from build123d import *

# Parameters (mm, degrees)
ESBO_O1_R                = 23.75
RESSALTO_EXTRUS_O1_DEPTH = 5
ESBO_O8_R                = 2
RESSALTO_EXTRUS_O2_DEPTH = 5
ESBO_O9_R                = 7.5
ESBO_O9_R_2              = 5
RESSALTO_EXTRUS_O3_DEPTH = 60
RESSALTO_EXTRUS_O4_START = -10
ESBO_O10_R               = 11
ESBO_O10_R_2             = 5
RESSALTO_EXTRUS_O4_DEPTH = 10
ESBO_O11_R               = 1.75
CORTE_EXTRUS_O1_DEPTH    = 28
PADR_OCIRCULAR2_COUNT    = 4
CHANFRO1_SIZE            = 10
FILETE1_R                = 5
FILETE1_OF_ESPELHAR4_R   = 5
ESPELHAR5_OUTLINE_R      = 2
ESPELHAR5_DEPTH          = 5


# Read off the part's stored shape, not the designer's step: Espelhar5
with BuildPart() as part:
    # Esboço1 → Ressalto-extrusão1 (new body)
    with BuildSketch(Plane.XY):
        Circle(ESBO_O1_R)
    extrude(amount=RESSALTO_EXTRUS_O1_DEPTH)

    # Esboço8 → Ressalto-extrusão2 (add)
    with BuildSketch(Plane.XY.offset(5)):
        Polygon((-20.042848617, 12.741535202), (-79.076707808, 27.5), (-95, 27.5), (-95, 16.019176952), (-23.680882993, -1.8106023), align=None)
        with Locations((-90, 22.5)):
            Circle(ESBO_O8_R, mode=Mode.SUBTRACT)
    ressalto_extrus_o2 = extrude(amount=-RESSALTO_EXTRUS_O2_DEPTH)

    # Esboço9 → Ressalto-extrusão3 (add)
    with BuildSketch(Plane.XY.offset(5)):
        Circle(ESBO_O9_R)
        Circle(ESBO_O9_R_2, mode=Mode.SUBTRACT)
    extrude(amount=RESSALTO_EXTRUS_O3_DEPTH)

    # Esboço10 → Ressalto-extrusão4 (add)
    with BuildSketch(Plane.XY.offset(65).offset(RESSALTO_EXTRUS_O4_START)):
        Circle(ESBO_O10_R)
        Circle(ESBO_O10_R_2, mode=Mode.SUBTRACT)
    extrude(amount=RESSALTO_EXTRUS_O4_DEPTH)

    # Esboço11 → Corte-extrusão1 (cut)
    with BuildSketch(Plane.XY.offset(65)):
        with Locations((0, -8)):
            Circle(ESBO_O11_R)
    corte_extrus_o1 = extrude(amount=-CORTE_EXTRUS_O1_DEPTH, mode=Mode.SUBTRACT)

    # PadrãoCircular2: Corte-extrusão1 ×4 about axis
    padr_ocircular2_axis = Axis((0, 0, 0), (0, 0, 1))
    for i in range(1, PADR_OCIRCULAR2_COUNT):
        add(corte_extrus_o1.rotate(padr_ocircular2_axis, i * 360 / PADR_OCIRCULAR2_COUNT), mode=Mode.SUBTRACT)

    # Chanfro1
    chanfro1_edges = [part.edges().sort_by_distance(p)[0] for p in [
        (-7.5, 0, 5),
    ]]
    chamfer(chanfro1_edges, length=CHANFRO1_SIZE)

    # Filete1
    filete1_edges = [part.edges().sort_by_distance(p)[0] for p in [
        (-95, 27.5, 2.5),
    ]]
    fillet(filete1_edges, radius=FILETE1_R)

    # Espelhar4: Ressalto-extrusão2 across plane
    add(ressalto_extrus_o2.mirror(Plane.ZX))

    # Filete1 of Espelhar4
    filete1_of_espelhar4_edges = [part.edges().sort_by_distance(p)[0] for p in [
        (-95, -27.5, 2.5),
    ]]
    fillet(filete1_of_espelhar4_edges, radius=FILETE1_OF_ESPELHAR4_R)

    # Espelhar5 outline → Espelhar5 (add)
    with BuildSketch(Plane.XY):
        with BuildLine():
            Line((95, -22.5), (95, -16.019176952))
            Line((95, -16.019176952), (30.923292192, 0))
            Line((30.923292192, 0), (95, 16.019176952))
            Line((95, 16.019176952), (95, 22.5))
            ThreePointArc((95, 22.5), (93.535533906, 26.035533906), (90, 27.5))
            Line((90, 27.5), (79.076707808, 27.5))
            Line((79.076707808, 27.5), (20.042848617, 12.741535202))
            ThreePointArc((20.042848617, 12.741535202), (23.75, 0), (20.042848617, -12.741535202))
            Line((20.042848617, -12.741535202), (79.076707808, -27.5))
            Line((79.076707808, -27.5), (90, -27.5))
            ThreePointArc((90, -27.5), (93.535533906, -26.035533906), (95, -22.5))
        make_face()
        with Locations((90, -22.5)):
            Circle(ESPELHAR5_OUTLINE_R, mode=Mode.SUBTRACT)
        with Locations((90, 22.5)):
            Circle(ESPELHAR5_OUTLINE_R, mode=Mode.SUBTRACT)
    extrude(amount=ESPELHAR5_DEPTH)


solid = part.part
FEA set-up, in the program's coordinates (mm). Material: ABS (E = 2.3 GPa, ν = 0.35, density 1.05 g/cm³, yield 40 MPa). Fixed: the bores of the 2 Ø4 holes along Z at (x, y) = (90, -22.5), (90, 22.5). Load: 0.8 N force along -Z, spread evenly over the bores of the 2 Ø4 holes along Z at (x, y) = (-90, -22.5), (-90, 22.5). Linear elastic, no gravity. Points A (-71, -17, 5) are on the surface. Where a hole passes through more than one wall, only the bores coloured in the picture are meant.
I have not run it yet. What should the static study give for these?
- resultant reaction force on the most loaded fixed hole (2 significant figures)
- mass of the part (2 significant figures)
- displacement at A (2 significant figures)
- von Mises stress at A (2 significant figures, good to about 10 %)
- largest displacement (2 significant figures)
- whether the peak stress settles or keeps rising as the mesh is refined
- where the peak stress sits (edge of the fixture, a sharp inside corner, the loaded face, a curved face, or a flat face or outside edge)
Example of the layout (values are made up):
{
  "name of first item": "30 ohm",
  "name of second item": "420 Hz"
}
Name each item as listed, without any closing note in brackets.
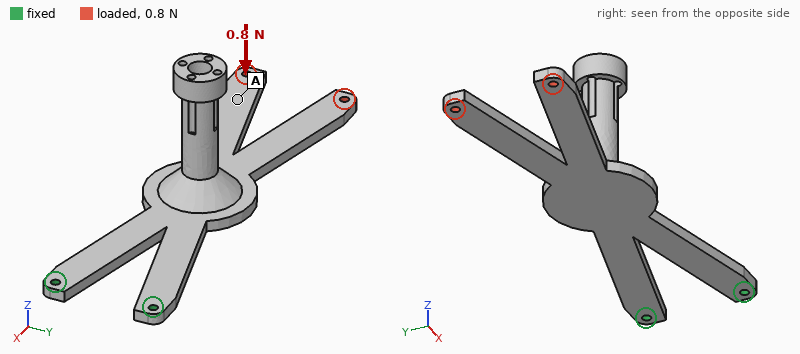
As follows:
{
  "resultant reaction force on the most loaded fixed hole": "0.40 N",
  "mass of the part": "43 g",
  "displacement at A": "1.7 mm",
  "von Mises stress at A": "0.13 MPa",
  "largest displacement": "2.1 mm",
  "whether the peak stress settles or keeps rising as the mesh is refined": "keeps rising",
  "where the peak stress sits": "edge of the fixture"
}
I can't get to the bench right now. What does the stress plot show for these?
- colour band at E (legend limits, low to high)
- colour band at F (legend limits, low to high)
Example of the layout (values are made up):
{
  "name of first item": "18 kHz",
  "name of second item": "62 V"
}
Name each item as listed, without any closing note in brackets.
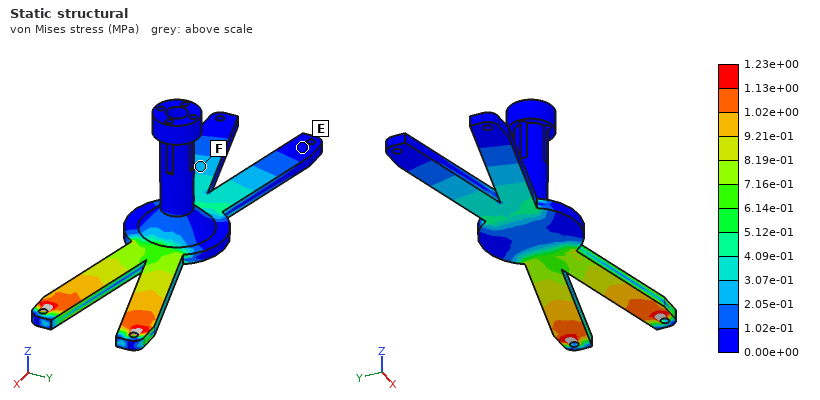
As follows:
{
  "colour band at E": "0.00e+00 to 1.02e-01 MPa",
  "colour band at F": "2.05e-01 to 3.07e-01 MPa"
}
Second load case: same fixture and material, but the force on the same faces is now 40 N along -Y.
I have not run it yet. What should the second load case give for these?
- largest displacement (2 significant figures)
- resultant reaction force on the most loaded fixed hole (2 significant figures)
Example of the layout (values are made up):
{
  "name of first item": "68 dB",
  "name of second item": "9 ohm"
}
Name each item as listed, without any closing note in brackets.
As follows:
{
  "largest displacement": "2.3 mm",
  "resultant reaction force on the most loaded fixed hole": "170 N"
}
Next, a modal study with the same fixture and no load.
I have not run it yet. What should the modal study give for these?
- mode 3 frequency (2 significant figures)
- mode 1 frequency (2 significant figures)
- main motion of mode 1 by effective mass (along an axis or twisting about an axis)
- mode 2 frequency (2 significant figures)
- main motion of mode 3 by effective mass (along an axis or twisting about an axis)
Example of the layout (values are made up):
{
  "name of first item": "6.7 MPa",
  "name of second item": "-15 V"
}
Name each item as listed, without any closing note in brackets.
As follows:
{
  "mode 3 frequency": "200 Hz",
  "mode 1 frequency": "32 Hz",
  "main motion of mode 1 by effective mass": "along Z",
  "mode 2 frequency": "130 Hz",
  "main motion of mode 3 by effective mass": "along Z"
}
